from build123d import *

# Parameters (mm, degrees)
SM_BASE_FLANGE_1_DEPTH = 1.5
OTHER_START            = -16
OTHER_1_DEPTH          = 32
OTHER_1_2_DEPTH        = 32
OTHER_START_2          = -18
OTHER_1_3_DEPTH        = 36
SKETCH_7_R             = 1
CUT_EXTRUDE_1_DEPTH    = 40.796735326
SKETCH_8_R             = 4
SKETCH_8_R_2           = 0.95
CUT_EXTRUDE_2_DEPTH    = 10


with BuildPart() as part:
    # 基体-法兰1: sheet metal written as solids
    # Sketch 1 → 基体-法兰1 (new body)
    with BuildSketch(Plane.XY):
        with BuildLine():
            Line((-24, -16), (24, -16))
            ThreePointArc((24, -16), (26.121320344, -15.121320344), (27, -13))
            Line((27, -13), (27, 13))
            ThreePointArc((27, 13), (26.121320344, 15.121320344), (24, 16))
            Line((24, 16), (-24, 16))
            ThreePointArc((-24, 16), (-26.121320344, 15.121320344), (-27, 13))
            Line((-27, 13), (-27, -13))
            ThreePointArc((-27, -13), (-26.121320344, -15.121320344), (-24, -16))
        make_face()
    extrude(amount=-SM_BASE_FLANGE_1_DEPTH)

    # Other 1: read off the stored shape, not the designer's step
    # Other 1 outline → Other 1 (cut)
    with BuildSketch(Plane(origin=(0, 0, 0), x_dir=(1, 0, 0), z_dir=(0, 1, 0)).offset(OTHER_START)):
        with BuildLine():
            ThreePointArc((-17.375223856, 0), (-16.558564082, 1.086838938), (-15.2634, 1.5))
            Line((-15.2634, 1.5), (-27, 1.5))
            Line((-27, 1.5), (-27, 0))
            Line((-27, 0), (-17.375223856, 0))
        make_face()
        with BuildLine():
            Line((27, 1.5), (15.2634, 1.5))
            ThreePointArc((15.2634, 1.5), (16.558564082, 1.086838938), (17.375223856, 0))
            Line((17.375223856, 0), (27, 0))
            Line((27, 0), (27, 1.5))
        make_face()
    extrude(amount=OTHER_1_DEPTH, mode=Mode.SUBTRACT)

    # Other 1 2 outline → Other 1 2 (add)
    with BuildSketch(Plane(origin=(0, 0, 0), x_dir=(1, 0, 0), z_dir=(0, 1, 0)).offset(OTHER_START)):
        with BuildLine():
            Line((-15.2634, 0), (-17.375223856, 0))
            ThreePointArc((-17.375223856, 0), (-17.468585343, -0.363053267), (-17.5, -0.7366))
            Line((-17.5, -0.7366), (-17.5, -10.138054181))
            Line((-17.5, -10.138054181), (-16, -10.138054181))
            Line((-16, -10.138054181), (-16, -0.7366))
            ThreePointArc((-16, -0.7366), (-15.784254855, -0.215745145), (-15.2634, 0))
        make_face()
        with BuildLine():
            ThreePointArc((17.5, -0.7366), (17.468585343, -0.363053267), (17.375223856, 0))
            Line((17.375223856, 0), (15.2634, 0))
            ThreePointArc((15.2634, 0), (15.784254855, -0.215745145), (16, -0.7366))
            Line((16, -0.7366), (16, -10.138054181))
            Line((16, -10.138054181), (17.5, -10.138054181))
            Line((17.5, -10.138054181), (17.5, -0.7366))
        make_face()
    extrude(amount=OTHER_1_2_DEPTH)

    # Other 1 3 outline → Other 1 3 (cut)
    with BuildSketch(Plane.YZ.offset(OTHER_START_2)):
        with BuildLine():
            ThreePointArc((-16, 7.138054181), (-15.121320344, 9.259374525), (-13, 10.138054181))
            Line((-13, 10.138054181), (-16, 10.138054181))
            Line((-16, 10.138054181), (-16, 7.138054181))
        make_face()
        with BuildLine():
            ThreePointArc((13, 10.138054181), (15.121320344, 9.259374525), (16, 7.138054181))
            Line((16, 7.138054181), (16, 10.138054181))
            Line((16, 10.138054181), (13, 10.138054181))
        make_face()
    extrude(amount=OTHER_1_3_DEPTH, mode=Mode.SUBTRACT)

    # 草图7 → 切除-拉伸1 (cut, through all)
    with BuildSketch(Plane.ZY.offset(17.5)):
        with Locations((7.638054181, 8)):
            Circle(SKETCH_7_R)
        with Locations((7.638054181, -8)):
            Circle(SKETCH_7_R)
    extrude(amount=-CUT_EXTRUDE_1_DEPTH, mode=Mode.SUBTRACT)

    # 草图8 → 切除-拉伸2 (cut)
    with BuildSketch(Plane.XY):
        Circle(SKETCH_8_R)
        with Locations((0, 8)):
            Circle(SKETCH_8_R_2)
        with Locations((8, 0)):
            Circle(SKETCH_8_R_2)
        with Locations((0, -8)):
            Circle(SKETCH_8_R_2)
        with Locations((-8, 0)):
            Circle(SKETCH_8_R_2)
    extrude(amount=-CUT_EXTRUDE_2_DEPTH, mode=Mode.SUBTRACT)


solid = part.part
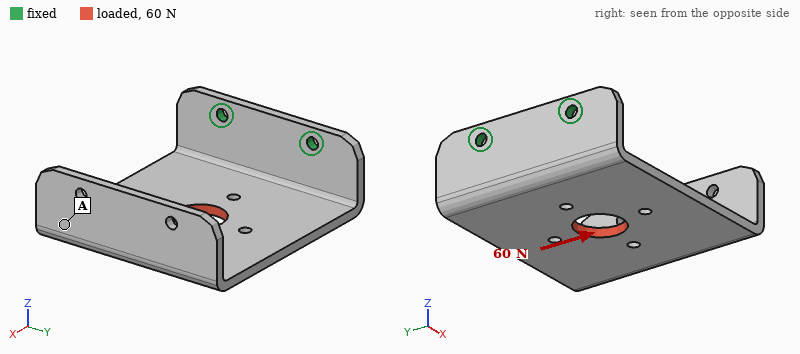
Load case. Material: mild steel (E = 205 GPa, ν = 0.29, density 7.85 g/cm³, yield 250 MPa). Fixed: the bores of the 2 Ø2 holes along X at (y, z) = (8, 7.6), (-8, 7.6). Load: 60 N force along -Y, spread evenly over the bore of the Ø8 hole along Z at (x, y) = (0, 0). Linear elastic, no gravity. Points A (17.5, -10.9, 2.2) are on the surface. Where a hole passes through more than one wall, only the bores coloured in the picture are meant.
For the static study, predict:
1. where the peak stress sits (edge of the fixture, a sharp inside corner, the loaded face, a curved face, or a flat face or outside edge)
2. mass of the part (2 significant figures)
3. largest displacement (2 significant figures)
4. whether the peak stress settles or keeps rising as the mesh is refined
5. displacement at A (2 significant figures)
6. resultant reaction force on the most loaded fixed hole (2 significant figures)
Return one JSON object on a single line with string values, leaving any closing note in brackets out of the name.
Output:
{"where the peak stress sits": "edge of the fixture", "mass of the part": "19 g", "largest displacement": "42 µm", "whether the peak stress settles or keeps rising as the mesh is refined": "keeps rising", "displacement at A": "35 µm", "resultant reaction force on the most loaded fixed hole": "68 N"}
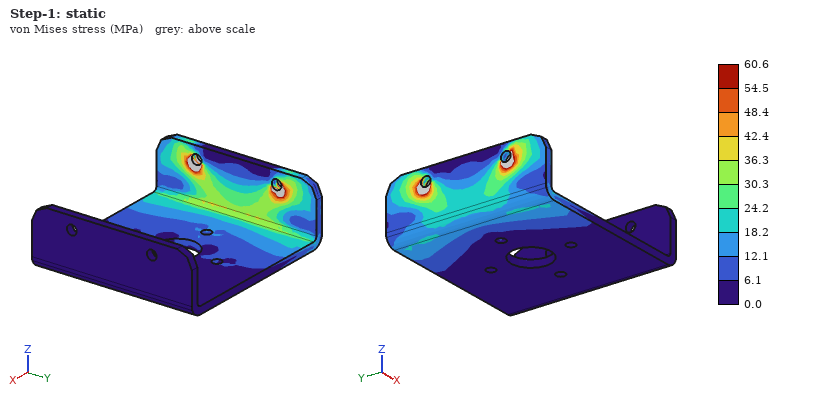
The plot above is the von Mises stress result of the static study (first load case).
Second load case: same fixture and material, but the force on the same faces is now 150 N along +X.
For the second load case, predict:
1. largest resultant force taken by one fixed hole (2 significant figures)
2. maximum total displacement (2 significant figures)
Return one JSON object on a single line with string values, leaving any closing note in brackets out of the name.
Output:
{"largest resultant force taken by one fixed hole": "75 N", "maximum total displacement": "0.12 mm"}
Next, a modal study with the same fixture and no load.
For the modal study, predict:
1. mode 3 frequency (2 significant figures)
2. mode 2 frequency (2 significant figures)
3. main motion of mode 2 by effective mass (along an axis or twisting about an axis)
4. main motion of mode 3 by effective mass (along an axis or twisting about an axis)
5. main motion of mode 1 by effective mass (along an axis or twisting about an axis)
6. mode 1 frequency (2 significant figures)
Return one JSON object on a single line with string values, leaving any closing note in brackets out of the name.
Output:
{"mode 3 frequency": "2300 Hz", "mode 2 frequency": "1300 Hz", "main motion of mode 2 by effective mass": "along Y", "main motion of mode 3 by effective mass": "along Y", "main motion of mode 1 by effective mass": "along Z", "mode 1 frequency": "540 Hz"}
